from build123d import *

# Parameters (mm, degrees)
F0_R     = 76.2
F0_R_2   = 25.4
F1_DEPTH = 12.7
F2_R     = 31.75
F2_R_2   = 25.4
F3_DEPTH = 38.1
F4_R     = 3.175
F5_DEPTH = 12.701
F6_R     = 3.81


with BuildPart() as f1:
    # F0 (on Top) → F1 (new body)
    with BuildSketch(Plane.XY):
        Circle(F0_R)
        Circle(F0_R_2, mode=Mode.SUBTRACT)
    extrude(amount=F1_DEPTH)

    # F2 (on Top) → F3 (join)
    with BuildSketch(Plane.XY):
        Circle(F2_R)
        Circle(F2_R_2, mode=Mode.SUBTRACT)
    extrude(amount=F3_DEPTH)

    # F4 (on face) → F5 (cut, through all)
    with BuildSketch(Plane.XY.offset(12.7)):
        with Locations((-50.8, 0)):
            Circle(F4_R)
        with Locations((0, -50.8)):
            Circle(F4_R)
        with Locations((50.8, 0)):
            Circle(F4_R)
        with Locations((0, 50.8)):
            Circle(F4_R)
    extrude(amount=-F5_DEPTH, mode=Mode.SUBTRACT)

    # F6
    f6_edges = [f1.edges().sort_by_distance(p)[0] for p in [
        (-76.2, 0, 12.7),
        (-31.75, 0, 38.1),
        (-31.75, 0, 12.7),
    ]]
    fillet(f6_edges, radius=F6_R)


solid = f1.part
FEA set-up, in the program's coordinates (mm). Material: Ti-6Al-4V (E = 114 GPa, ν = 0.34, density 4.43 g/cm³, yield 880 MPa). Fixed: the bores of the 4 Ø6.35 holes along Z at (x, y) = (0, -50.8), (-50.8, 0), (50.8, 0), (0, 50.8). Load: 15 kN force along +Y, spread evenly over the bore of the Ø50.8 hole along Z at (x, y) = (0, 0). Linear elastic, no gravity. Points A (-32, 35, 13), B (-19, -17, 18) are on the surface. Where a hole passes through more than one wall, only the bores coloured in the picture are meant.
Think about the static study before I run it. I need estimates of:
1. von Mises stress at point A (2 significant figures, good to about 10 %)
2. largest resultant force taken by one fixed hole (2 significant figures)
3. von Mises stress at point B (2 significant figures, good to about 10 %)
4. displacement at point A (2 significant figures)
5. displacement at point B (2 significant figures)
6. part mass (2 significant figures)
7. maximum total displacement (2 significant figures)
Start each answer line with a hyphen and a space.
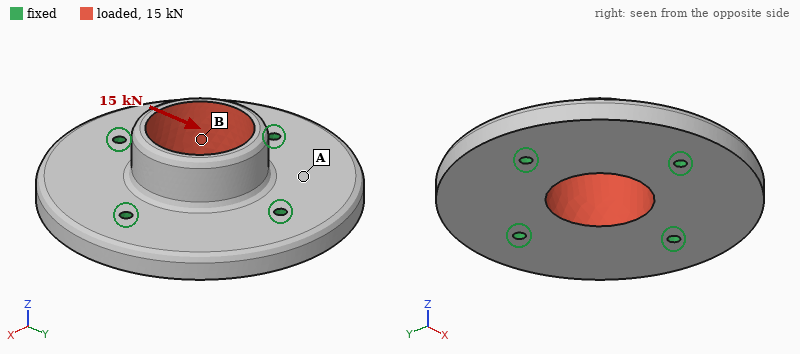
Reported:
- 5.3 MPa
- 4.6 kN
- 17 MPa
- 3.5 µm
- 6.1 µm
- 1.0 kg
- 15 µm
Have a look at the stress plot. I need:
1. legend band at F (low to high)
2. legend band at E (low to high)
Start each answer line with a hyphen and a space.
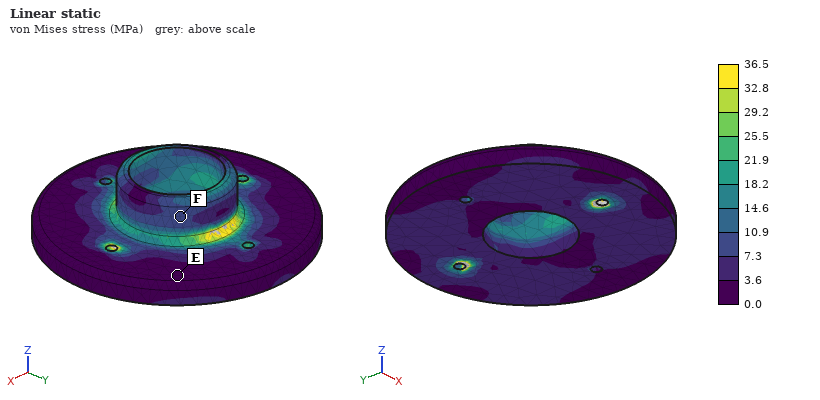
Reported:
- 7.3 to 10.9 MPa
- 0.0 to 3.6 MPa
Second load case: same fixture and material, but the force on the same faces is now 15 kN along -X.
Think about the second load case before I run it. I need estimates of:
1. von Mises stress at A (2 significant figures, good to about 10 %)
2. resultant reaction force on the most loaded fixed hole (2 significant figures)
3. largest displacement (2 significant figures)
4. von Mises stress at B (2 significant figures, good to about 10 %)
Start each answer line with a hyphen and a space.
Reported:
- 4.8 MPa
- 4.6 kN
- 15 µm
- 16 MPa
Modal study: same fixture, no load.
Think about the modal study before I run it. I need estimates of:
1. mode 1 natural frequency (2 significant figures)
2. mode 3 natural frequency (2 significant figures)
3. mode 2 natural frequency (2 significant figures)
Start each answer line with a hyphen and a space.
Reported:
- 4900 Hz
- 5700 Hz
- 5700 Hz
